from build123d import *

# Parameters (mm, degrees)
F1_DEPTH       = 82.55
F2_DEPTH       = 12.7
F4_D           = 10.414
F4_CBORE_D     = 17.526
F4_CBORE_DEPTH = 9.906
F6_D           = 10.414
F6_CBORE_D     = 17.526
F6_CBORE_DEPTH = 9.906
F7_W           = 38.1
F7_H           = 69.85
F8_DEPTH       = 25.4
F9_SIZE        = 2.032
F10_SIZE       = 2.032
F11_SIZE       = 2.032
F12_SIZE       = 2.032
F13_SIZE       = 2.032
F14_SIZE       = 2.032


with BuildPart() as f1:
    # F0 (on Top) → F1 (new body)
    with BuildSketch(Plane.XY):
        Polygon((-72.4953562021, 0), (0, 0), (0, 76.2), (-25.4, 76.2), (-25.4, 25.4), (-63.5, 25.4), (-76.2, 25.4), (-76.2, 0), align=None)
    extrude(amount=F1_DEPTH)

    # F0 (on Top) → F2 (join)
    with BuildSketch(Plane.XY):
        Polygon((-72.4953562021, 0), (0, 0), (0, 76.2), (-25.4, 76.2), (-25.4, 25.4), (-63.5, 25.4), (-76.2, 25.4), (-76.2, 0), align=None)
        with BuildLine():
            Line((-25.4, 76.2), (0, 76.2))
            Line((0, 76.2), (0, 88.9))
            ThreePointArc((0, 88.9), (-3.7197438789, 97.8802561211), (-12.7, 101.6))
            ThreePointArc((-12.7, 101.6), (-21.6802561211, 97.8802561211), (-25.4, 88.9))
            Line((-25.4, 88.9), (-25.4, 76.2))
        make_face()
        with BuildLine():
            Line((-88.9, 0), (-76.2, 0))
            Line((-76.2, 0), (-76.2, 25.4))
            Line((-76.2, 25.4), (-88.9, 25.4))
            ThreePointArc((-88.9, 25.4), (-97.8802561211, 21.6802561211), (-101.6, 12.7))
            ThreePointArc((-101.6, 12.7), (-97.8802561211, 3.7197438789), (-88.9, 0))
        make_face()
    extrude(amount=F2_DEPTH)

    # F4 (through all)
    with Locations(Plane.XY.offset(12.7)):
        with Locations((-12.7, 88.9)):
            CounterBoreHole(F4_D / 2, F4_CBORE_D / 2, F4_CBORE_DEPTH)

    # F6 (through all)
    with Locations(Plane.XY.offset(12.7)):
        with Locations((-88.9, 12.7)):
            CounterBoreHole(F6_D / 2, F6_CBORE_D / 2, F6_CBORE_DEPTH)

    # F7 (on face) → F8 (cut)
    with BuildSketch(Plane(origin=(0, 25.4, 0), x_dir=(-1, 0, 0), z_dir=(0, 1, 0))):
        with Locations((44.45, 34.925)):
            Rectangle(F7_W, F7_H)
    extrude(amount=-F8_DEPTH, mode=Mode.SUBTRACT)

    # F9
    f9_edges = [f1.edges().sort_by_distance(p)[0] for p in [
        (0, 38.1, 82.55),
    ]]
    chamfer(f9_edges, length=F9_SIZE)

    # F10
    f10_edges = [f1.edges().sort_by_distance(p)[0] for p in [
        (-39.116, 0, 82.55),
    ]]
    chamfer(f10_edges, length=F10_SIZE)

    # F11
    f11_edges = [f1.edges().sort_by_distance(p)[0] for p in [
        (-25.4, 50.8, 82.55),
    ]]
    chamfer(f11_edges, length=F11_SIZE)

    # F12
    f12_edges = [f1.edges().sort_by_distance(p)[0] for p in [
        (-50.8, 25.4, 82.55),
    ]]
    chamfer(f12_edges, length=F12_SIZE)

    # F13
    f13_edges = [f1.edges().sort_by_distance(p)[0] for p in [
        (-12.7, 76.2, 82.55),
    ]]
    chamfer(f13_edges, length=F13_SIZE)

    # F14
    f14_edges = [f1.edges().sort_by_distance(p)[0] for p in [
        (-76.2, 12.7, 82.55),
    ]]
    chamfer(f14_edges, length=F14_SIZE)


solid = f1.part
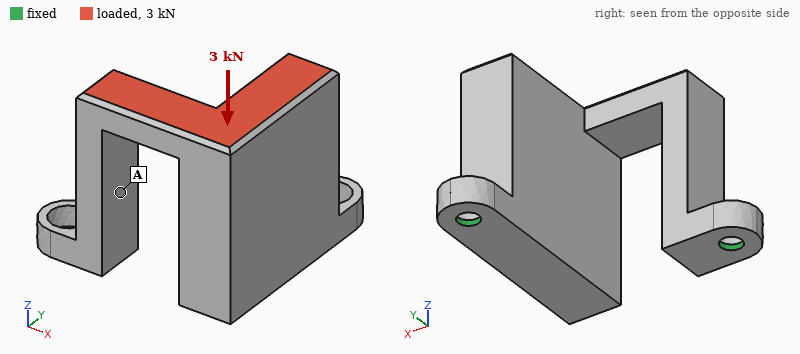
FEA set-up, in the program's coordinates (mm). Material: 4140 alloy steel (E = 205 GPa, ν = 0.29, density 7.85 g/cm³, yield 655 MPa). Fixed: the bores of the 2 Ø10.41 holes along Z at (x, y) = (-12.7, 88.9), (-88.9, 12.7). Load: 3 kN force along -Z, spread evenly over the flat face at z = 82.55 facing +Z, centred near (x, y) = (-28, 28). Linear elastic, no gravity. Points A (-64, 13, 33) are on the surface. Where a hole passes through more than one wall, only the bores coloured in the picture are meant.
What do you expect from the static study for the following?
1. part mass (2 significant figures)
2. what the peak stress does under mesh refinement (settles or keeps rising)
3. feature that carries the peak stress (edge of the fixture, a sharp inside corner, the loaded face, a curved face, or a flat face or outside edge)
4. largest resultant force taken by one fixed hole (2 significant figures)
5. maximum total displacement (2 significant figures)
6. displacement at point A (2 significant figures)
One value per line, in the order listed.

1.6 kg
keeps rising
edge of the fixture
1.6 kN
0.33 mm
0.094 mm
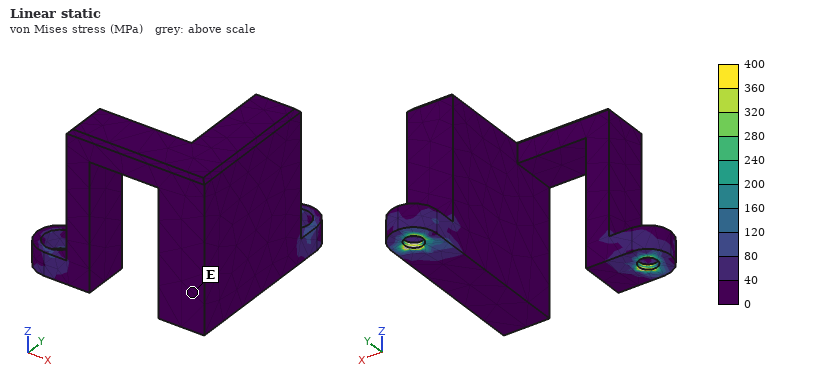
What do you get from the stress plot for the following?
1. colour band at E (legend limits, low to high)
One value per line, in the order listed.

0 to 40 MPa
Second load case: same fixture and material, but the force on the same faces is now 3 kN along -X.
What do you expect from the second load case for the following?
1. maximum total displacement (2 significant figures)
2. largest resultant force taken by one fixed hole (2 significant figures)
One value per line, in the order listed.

0.62 mm
2.3 kN
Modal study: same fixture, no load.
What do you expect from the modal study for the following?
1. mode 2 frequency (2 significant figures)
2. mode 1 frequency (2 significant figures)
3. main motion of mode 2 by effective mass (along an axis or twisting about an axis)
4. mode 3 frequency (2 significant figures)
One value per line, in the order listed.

1000 Hz
370 Hz
along X
1600 Hz
